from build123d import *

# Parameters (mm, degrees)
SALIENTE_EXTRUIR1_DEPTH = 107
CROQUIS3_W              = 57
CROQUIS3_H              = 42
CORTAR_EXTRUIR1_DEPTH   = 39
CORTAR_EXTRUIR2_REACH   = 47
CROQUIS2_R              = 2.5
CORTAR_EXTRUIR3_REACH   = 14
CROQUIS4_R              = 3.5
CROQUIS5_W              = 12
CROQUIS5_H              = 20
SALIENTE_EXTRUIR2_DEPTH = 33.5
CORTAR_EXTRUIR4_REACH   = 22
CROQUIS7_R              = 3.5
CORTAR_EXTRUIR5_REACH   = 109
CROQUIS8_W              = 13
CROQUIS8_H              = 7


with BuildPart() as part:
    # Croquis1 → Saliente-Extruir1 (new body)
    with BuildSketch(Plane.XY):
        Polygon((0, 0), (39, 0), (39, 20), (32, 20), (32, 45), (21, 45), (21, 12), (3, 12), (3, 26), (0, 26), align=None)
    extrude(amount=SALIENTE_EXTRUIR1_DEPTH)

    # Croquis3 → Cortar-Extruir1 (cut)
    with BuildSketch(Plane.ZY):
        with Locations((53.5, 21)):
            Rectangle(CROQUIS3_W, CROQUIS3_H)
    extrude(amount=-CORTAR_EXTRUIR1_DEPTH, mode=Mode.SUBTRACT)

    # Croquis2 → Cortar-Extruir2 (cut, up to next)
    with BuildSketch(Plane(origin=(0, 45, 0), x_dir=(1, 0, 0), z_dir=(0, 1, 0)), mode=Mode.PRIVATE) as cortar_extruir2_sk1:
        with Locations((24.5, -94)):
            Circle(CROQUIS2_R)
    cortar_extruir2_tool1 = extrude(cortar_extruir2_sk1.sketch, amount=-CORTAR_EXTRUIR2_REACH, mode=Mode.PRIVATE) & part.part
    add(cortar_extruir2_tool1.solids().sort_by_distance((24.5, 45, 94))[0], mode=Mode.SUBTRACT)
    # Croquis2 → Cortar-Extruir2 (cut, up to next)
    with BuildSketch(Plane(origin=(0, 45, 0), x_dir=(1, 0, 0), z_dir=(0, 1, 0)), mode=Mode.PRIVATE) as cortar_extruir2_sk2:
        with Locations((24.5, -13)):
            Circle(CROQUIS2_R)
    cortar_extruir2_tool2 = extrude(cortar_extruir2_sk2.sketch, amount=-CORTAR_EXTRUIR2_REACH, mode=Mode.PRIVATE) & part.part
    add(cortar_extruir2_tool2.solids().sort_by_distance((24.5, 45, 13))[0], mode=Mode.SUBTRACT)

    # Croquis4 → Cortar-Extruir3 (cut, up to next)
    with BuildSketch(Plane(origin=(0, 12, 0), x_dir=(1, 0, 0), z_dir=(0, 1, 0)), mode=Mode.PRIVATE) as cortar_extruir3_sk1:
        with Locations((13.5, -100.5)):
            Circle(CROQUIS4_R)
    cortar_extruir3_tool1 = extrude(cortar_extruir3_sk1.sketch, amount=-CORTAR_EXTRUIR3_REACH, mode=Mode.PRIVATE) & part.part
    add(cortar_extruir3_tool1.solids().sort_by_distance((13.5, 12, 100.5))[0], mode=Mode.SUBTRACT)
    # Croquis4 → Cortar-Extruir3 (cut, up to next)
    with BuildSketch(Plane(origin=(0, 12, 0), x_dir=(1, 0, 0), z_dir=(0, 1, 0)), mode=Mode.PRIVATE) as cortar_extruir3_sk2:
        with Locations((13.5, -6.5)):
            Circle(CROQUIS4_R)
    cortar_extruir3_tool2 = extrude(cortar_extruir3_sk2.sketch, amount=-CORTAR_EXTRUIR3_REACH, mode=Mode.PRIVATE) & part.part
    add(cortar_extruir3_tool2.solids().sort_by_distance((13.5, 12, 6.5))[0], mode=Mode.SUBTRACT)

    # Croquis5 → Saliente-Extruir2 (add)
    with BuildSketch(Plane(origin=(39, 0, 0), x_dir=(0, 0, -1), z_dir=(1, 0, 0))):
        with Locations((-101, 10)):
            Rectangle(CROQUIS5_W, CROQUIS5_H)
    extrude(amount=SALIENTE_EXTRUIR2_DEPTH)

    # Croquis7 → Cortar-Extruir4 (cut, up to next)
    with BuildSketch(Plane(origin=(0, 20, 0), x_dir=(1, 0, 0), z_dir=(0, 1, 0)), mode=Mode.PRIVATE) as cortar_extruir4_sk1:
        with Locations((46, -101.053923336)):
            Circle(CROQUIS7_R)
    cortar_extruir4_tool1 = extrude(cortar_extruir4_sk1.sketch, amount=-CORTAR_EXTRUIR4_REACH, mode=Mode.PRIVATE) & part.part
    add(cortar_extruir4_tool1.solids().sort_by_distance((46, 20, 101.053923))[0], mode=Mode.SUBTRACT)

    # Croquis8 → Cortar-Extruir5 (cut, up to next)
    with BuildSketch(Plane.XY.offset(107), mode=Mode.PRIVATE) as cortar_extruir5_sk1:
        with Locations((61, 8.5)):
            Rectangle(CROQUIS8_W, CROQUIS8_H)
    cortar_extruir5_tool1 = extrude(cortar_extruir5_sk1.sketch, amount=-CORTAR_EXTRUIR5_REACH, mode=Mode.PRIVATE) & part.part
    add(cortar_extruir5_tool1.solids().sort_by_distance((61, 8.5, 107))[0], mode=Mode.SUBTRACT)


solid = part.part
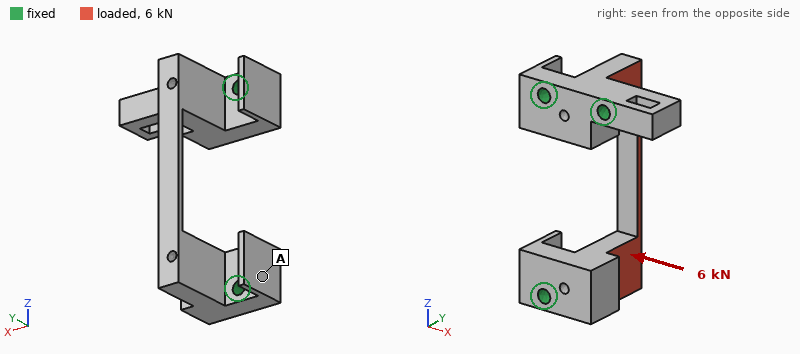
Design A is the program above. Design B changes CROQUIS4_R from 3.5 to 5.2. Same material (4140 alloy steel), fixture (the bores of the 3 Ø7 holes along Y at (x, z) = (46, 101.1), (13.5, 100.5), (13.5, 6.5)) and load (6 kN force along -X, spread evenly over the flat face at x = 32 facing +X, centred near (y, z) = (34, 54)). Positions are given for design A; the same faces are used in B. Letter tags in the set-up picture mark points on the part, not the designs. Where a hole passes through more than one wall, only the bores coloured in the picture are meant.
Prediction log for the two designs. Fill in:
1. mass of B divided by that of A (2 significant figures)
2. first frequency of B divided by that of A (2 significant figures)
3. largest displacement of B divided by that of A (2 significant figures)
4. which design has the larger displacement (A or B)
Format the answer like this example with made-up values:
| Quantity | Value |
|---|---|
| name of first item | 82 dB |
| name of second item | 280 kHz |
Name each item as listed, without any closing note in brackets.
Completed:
| Quantity | Value |
|---|---|
| mass of B divided by that of A | 0.98 |
| first frequency of B divided by that of A | 1.1 |
| largest displacement of B divided by that of A | 0.89 |
| which design has the larger displacement | A |
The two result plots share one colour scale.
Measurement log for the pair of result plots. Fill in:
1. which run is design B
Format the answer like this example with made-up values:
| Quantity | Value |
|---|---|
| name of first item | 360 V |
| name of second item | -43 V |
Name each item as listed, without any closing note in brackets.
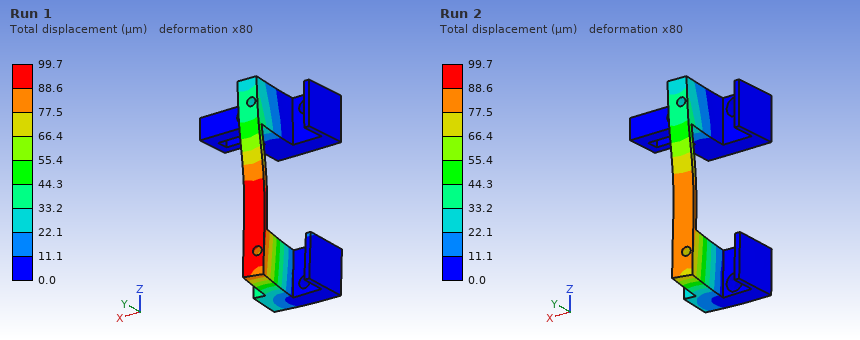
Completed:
| Quantity | Value |
|---|---|
| which run is design B | Run 2 |
